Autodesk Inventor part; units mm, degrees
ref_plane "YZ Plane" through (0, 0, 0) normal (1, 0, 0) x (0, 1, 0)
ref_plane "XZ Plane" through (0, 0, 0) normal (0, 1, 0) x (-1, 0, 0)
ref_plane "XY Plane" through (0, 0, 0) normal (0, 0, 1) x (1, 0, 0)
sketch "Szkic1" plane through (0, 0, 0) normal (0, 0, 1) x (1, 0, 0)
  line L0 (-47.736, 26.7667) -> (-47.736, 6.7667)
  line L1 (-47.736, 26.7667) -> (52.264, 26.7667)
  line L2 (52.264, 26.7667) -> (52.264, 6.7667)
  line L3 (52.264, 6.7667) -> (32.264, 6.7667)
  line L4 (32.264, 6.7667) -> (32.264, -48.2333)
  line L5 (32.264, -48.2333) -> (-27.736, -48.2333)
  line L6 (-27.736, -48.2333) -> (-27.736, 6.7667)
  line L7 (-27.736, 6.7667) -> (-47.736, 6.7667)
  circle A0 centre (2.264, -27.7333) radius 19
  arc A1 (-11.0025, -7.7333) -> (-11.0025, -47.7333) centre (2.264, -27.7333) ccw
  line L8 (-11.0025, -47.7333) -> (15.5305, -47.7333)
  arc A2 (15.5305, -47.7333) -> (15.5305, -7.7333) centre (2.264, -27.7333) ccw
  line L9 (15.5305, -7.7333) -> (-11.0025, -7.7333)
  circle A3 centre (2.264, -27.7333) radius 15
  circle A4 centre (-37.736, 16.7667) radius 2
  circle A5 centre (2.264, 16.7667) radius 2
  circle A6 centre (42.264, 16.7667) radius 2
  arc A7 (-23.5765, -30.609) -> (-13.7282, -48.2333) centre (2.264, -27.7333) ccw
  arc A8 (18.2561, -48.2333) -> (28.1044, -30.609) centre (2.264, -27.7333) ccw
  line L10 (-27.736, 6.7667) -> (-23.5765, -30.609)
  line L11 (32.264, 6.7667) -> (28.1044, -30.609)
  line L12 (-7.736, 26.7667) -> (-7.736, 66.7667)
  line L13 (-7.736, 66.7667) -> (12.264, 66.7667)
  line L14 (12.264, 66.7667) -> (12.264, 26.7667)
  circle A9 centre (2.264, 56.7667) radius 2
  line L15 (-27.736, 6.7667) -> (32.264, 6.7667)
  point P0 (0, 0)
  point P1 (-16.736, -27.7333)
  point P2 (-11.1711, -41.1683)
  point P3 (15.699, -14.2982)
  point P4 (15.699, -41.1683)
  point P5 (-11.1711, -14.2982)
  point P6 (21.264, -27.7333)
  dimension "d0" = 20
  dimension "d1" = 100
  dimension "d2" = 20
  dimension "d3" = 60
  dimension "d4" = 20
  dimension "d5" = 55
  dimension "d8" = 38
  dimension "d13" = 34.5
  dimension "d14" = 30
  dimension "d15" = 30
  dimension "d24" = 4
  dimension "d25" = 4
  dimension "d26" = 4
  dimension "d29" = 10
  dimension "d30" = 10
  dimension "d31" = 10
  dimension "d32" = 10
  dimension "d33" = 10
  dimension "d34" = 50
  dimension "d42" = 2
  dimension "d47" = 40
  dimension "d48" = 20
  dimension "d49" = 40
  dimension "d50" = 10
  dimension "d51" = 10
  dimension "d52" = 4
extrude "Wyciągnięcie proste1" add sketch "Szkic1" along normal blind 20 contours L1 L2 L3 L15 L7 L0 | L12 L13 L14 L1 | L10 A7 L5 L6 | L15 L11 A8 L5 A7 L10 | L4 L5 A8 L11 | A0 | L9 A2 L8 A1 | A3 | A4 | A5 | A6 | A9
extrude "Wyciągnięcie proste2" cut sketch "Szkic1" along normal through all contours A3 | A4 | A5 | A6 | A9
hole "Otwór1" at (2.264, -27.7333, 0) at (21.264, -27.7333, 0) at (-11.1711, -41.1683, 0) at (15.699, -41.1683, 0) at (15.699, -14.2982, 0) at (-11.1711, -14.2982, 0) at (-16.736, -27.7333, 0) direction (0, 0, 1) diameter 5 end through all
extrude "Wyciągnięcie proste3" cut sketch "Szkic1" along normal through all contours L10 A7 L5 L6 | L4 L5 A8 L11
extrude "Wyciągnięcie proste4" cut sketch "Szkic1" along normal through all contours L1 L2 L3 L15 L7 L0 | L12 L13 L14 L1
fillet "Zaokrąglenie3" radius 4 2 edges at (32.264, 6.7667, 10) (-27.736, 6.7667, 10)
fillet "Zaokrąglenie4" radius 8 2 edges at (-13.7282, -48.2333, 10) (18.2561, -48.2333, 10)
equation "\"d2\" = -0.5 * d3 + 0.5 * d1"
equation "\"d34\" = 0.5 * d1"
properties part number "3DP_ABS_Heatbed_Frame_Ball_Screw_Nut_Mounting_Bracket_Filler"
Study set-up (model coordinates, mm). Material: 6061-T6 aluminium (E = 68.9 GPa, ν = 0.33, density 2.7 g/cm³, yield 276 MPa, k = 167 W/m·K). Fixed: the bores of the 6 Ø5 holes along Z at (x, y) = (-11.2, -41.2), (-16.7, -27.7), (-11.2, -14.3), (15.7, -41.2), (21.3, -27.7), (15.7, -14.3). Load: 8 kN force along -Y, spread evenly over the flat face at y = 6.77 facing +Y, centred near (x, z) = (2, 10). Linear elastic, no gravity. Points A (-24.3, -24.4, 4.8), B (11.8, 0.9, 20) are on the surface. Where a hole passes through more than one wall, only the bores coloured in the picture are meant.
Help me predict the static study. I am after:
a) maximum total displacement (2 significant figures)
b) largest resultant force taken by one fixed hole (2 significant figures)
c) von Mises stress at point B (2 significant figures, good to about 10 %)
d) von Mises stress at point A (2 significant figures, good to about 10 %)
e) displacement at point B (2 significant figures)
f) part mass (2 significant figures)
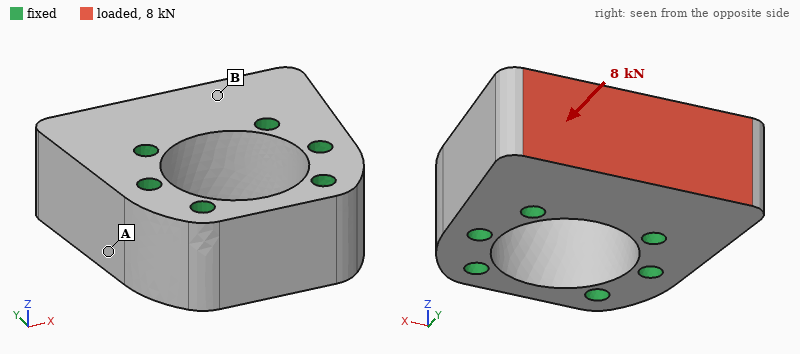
3.4 µm
3.4 kN
8.4 MPa
3.3 MPa
2.5 µm
110 g
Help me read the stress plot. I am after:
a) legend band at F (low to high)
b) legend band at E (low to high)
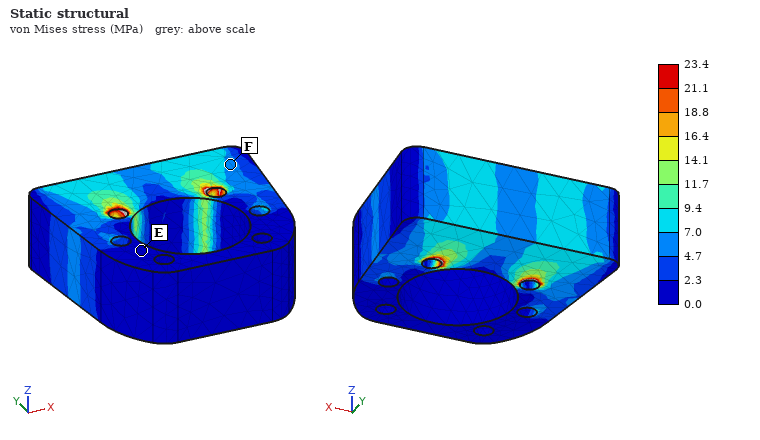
4.7 to 7.0 MPa
0.0 to 2.3 MPa
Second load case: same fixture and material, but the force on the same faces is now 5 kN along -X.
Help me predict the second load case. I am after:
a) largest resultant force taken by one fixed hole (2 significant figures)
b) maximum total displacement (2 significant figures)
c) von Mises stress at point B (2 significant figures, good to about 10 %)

3.2 kN
7.7 µm
10 MPa
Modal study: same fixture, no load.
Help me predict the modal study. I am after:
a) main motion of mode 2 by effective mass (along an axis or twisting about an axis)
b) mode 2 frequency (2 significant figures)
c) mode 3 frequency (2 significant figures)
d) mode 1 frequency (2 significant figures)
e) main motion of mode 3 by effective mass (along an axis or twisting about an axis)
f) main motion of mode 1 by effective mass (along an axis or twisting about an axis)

twisting about Y
24 kHz
26 kHz
20 kHz
along X
along Z
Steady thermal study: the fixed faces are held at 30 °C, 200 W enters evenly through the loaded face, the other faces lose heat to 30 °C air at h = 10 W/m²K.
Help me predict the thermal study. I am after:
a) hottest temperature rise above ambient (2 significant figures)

27 K
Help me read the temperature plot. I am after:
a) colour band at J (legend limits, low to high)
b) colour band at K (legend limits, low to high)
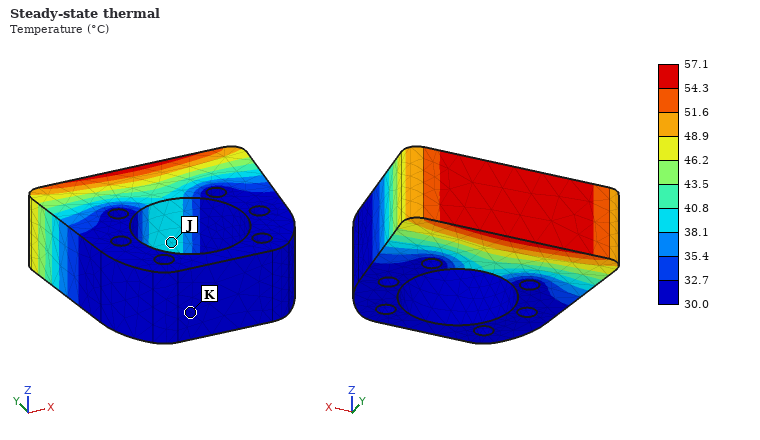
38.1 to 40.8 °C
30.0 to 32.7 °C
